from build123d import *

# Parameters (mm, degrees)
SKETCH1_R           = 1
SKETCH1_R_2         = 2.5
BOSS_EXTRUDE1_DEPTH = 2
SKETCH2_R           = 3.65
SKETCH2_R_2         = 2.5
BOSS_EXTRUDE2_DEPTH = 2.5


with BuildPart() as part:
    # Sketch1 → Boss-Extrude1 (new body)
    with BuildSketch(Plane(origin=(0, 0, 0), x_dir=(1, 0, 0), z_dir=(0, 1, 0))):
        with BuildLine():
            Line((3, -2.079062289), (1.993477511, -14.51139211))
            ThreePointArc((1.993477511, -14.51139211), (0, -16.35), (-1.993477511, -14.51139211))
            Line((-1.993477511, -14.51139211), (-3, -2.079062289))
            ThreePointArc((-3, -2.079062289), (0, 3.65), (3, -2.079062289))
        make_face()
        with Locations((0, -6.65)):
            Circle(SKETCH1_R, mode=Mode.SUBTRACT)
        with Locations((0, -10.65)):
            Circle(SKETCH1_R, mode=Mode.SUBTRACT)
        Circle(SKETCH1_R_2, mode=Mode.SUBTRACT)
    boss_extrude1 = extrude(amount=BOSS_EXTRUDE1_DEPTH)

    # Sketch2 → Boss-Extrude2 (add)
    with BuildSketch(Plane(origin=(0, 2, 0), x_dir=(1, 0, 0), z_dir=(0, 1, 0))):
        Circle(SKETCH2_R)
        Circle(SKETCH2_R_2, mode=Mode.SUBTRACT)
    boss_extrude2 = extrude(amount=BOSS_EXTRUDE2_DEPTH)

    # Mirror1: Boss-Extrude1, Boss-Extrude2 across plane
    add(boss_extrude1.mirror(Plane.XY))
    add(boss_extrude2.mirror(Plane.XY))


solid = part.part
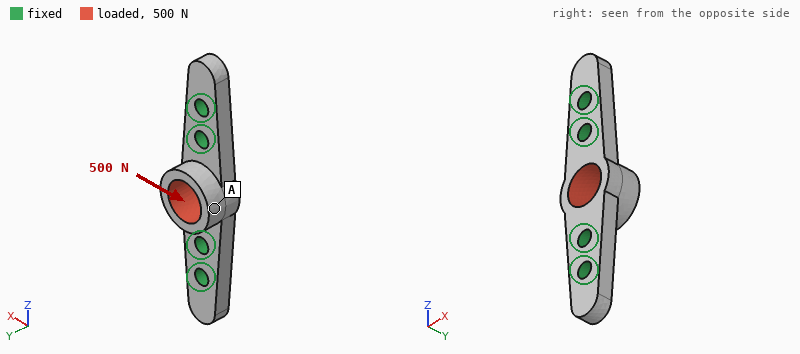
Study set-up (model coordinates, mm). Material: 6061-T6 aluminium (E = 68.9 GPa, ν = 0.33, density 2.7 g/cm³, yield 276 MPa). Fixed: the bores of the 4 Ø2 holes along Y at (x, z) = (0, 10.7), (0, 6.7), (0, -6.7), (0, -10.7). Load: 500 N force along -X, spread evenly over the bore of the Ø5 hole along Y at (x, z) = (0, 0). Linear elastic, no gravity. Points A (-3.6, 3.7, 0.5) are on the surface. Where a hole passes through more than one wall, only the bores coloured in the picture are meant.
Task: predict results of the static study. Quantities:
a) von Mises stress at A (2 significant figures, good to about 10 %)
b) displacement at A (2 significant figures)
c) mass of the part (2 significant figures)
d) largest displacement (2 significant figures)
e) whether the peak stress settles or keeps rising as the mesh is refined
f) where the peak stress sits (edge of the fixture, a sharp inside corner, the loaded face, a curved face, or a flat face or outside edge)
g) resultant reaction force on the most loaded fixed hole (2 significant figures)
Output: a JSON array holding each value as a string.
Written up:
["21 MPa", "20 µm", "0.86 g", "22 µm", "keeps rising", "edge of the fixture", "290 N"]
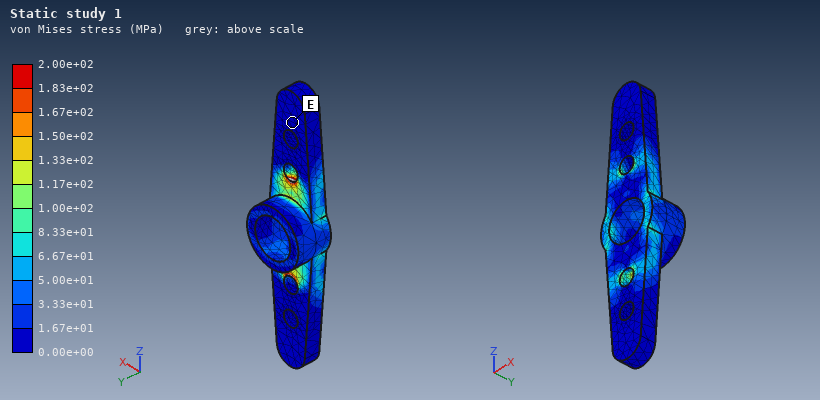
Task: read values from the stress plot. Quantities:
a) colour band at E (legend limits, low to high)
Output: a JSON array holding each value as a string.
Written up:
["0.00e+00 to 1.67e+01 MPa"]
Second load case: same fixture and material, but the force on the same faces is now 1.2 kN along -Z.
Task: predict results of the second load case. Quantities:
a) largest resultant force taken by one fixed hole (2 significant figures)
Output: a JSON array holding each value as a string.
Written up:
["560 N"]
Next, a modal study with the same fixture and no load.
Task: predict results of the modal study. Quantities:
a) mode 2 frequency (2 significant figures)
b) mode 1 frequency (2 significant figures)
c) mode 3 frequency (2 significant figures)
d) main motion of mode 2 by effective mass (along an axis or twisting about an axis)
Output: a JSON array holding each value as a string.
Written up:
["55 kHz", "44 kHz", "67 kHz", "along Y"]
